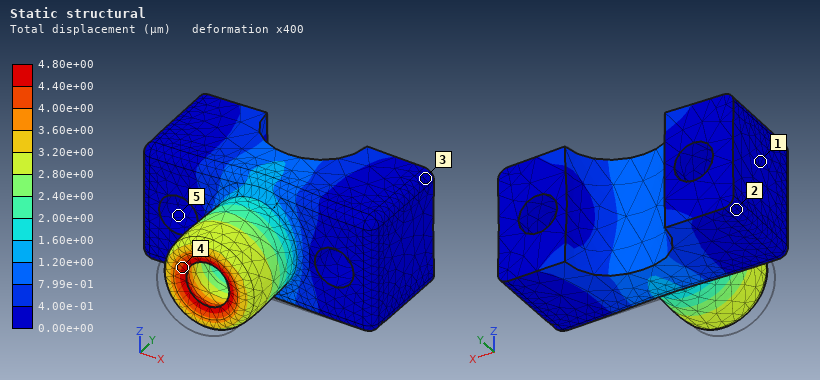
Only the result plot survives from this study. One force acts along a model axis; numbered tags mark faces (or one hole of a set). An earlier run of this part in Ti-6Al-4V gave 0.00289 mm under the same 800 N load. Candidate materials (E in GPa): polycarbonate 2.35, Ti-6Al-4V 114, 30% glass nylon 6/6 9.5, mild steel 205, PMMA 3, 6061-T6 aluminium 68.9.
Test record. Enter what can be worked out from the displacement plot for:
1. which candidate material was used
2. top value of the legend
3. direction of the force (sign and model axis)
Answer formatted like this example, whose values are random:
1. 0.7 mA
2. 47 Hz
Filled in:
1. 6061-T6 aluminium
2. 4.80e+00 µm
3. +Y
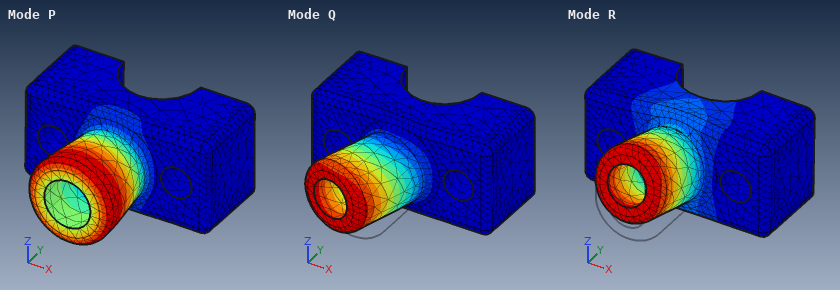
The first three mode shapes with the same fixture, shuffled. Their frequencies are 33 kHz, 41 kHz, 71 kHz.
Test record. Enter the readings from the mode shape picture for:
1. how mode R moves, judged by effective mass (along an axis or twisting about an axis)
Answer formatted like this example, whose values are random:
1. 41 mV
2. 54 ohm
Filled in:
1. along Z
